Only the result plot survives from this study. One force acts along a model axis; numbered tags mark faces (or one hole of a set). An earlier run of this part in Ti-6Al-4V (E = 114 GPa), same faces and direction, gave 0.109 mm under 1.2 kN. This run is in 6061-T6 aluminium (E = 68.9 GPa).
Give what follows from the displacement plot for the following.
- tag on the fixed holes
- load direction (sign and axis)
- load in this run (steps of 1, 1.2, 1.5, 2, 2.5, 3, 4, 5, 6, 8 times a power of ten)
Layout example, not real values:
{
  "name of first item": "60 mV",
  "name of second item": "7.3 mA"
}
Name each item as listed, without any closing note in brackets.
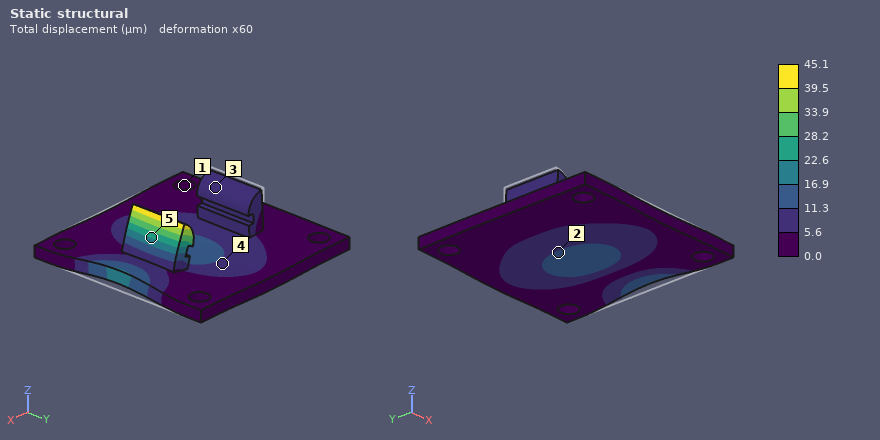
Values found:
{
  "tag on the fixed holes": "1",
  "load direction": "-X",
  "load in this run": "300 N"
}
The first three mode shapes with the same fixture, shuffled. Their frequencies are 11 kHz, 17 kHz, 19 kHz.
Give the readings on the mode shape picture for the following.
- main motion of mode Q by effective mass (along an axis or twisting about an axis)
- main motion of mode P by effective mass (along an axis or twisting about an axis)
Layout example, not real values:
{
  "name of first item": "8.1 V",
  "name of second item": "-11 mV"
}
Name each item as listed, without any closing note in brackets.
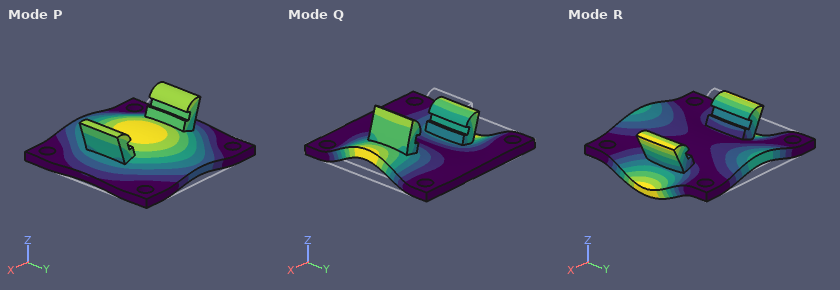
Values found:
{
  "main motion of mode Q by effective mass": "twisting about Y",
  "main motion of mode P by effective mass": "along Z"
}
